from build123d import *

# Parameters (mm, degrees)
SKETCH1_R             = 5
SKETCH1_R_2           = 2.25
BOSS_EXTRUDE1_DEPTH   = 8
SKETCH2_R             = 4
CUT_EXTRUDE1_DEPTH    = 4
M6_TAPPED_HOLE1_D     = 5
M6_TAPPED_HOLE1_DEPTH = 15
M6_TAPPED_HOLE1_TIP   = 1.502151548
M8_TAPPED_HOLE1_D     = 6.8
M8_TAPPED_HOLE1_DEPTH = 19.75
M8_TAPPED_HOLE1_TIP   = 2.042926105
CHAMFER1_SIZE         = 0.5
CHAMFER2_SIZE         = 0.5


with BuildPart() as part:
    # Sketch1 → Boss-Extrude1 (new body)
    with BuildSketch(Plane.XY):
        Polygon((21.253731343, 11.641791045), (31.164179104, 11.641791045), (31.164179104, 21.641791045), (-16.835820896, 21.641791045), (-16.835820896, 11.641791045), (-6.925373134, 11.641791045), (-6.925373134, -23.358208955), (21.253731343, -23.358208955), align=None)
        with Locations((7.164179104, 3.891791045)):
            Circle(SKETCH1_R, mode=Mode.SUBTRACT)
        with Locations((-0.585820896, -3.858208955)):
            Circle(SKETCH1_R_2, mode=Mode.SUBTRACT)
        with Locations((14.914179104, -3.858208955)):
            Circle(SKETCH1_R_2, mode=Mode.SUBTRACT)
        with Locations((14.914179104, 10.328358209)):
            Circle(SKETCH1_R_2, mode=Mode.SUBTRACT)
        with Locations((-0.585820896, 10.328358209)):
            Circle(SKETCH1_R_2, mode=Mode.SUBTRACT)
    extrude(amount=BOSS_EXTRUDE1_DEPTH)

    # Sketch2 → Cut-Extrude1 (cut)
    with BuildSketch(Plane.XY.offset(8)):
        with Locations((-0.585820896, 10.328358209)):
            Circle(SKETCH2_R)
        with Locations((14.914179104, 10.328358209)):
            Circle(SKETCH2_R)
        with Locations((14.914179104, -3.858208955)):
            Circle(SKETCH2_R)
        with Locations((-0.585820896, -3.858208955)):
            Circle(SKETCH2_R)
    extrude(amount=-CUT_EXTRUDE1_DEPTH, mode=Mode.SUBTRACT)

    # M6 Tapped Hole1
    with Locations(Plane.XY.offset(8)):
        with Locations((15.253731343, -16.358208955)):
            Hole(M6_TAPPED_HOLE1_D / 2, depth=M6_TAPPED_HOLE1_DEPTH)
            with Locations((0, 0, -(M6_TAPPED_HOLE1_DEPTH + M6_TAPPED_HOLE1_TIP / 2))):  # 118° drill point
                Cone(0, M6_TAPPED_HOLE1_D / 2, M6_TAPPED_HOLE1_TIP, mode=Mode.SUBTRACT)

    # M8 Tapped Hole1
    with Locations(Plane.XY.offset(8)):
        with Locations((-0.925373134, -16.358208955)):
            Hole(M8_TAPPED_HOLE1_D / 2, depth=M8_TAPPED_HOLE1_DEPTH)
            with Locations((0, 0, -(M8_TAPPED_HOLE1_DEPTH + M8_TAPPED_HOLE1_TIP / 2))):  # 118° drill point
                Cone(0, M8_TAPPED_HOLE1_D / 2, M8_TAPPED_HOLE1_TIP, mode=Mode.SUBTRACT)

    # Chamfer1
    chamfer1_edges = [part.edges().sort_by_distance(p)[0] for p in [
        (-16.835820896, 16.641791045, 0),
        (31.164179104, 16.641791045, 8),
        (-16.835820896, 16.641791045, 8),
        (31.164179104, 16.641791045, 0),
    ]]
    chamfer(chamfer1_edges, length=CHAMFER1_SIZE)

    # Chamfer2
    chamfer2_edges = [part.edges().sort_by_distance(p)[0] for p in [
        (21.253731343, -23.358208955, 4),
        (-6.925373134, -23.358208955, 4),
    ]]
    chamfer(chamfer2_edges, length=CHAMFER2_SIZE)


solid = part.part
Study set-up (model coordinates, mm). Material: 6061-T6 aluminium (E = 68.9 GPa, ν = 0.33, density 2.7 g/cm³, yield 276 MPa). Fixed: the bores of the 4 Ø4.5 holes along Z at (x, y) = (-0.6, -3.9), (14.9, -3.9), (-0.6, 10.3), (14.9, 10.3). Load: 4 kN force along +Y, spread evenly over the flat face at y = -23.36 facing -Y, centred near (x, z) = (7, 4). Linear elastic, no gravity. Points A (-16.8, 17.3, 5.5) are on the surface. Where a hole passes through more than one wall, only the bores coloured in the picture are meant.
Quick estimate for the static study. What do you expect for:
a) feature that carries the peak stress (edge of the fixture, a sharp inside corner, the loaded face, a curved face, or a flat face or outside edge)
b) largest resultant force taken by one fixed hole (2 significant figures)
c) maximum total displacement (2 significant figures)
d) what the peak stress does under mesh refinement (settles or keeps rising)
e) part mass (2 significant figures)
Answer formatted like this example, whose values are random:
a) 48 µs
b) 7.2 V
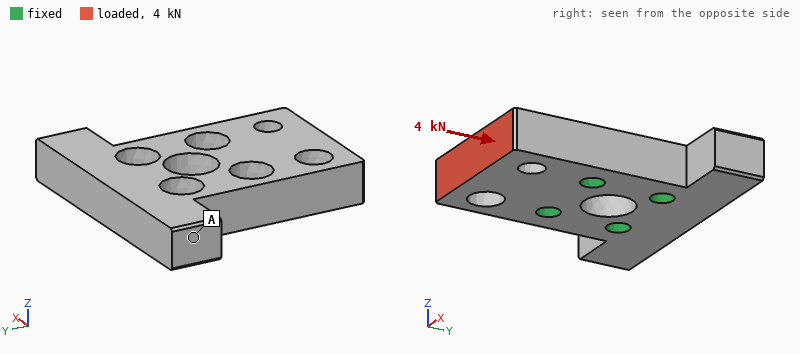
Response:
a) edge of the fixture
b) 1.7 kN
c) 23 µm
d) keeps rising
e) 26 g
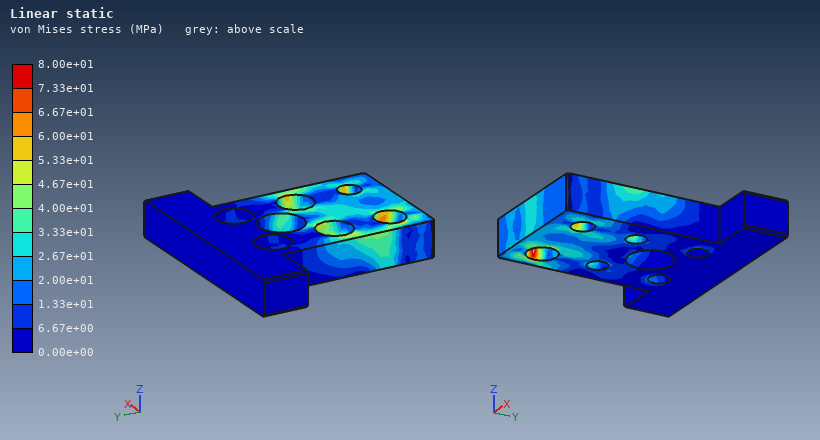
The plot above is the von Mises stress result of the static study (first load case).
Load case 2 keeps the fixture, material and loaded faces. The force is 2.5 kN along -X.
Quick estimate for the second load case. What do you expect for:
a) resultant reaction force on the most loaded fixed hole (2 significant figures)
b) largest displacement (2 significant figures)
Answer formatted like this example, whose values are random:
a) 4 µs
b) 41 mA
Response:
a) 2.5 kN
b) 30 µm
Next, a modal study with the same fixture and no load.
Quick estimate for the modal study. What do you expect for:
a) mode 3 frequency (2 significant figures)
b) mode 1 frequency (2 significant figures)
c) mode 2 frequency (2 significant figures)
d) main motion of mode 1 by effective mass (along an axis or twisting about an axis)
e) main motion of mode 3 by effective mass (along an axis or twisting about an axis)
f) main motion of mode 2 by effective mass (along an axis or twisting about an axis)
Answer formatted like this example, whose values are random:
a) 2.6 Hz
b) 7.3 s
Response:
a) 16 kHz
b) 11 kHz
c) 15 kHz
d) along Z
e) along Z
f) twisting about Y
